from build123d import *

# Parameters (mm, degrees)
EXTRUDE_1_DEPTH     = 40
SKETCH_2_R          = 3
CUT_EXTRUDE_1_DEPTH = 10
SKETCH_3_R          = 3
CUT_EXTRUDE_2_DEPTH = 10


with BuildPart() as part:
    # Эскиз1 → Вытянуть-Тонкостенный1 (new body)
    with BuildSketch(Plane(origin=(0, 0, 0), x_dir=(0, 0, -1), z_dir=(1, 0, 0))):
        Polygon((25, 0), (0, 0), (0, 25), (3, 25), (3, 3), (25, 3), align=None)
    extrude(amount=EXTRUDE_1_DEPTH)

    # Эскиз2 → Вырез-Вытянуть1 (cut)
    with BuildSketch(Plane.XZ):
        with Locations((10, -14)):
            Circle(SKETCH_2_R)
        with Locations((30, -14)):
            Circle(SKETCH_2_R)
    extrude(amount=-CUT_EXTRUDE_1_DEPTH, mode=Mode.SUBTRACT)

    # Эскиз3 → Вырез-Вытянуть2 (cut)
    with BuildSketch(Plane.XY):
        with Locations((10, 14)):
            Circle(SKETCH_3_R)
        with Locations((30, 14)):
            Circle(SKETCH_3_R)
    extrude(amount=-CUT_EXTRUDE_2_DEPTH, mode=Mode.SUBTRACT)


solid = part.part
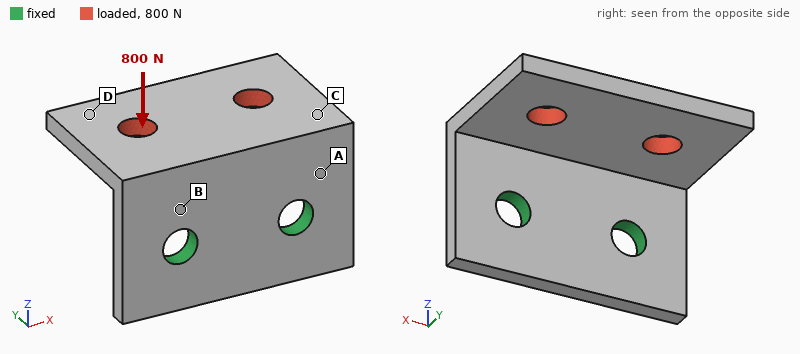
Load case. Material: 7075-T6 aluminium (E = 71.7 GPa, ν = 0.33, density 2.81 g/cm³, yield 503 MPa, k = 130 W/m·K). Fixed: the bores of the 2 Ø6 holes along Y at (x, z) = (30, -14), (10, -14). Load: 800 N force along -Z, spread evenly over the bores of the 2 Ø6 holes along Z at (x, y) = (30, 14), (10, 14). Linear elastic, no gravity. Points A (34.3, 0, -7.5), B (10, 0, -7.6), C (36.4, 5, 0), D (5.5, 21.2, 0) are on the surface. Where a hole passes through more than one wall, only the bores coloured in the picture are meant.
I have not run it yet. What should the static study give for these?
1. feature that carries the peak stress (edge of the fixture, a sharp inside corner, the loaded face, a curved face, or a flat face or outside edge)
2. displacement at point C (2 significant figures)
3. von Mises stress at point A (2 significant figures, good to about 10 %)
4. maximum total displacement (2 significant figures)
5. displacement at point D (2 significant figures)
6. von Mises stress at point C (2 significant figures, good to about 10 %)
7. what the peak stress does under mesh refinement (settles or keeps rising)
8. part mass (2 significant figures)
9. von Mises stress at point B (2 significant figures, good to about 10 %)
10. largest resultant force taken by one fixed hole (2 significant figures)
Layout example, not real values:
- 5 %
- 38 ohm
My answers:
- edge of the fixture
- 0.13 mm
- 140 MPa
- 0.54 mm
- 0.44 mm
- 110 MPa
- keeps rising
- 15 g
- 160 MPa
- 410 N
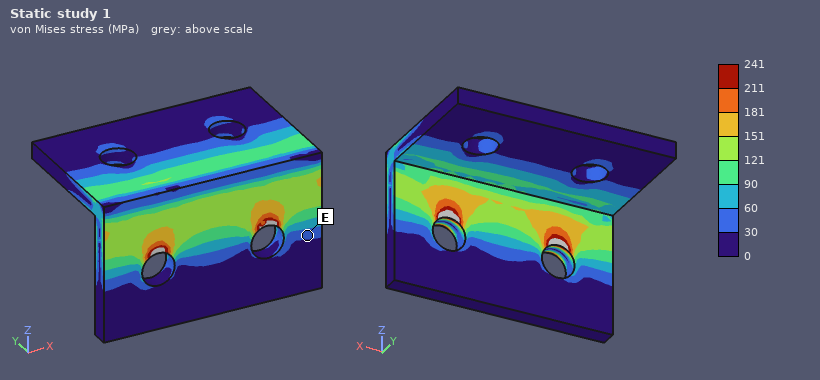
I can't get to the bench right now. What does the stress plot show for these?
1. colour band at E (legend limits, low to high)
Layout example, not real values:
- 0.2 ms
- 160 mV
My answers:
- 30 to 60 MPa
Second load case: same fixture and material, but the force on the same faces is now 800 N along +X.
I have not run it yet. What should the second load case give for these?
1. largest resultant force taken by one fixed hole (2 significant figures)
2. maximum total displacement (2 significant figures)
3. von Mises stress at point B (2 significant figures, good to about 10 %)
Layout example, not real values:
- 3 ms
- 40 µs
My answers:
- 670 N
- 0.11 mm
- 52 MPa
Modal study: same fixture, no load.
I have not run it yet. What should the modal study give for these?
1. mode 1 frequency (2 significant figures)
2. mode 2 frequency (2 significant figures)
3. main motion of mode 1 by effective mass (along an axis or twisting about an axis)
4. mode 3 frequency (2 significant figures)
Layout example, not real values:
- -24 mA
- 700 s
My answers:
- 2700 Hz
- 4900 Hz
- along Z
- 7500 Hz
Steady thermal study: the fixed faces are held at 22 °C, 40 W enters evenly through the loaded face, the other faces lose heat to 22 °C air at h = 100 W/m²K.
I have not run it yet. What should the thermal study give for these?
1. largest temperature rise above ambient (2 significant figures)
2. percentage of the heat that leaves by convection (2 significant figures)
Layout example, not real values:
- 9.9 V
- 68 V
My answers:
- 56 K
- 24 %
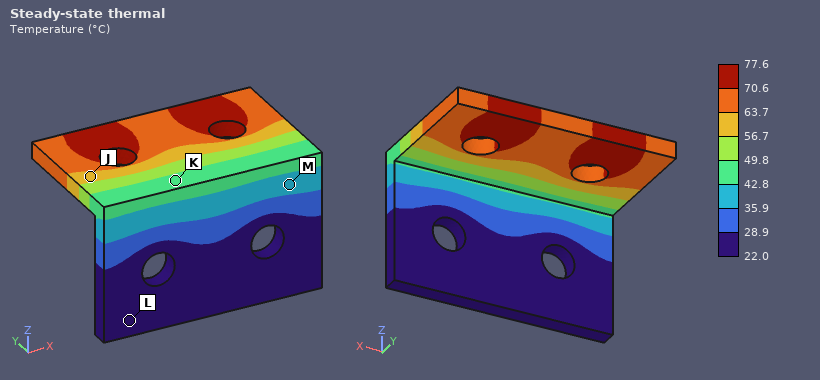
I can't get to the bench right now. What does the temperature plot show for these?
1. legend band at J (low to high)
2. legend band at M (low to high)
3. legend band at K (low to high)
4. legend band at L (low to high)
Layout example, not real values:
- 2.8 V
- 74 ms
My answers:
- 56.7 to 63.7 °C
- 35.9 to 42.8 °C
- 42.8 to 49.8 °C
- 22.0 to 28.9 °C
